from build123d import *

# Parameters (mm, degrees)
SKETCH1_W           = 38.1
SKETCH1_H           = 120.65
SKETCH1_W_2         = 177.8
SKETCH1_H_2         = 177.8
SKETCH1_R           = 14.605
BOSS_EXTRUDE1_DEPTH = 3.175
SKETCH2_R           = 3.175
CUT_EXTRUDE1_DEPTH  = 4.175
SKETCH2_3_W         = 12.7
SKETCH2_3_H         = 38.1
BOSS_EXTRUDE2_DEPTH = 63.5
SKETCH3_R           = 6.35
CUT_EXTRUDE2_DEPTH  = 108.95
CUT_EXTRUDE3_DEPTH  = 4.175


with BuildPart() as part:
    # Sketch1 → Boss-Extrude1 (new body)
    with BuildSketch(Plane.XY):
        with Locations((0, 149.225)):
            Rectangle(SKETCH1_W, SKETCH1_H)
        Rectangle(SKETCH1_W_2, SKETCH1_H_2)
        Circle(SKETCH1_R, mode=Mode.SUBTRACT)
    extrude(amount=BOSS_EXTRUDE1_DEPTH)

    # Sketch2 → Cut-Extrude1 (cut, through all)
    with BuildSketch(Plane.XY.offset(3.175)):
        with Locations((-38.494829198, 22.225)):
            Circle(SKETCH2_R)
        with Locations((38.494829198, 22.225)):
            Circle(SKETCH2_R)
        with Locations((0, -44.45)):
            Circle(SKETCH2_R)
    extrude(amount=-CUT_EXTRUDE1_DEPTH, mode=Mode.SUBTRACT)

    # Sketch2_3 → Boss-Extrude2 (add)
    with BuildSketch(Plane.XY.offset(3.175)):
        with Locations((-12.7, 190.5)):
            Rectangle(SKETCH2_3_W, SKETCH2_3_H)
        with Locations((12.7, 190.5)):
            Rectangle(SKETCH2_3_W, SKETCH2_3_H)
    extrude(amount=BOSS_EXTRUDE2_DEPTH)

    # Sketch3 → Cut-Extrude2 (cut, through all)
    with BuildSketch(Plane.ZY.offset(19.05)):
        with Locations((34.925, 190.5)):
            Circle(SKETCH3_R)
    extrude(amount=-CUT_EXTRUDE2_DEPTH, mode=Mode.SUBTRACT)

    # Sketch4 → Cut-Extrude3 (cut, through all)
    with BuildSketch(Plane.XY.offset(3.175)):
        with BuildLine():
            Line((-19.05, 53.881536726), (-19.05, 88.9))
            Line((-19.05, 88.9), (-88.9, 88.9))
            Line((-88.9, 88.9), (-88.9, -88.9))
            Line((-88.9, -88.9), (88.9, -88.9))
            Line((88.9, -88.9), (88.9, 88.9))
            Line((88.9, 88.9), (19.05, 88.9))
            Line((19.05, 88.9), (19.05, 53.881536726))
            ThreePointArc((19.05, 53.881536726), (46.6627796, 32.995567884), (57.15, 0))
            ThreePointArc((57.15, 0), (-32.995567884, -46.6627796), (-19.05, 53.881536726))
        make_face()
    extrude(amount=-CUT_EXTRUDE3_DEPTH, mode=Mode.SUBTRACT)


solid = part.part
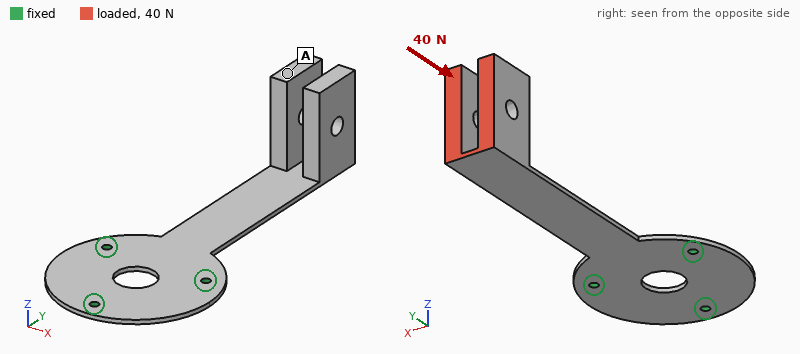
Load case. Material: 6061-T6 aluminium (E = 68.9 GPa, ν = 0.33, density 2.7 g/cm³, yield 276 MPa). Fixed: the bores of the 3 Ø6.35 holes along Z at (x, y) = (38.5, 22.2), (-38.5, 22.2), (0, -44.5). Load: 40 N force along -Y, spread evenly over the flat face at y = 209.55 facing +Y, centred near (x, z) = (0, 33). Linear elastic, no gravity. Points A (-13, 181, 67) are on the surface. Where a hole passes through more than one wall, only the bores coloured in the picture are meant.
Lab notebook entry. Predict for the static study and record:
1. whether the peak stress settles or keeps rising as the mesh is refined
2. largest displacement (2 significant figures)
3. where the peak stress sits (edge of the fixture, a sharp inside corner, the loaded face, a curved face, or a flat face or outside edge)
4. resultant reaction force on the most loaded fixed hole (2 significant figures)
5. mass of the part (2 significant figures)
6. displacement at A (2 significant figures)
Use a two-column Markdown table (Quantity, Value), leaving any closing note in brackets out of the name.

| Quantity | Value |
|---|---|
| whether the peak stress settles or keeps rising as the mesh is refined | keeps rising |
| largest displacement | 3.1 mm |
| where the peak stress sits | a sharp inside corner |
| resultant reaction force on the most loaded fixed hole | 20 N |
| mass of the part | 290 g |
| displacement at A | 2.5 mm |
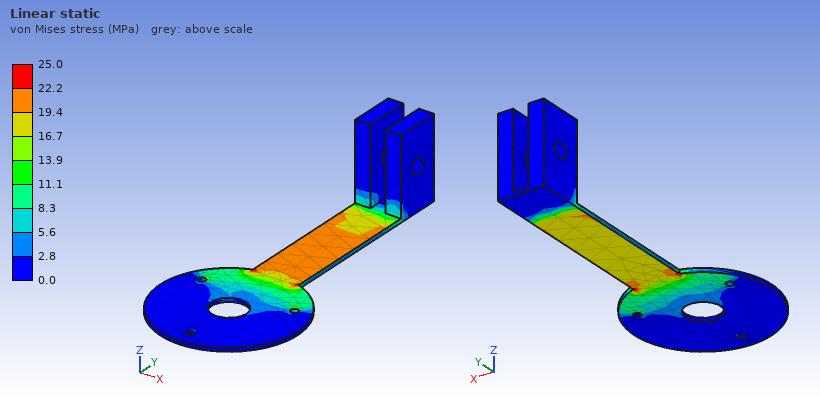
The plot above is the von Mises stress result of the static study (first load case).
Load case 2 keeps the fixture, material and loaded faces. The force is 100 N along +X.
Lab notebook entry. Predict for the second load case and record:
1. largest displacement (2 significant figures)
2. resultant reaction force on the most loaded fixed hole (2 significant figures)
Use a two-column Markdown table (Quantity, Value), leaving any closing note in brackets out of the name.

| Quantity | Value |
|---|---|
| largest displacement | 2.7 mm |
| resultant reaction force on the most loaded fixed hole | 250 N |
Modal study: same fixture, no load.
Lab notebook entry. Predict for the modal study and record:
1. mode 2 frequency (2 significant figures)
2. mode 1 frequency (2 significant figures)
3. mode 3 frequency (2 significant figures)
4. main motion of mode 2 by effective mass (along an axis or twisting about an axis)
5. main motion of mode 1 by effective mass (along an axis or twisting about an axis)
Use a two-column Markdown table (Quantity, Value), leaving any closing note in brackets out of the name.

| Quantity | Value |
|---|---|
| mode 2 frequency | 88 Hz |
| mode 1 frequency | 26 Hz |
| mode 3 frequency | 160 Hz |
| main motion of mode 2 by effective mass | along X |
| main motion of mode 1 by effective mass | along Z |
